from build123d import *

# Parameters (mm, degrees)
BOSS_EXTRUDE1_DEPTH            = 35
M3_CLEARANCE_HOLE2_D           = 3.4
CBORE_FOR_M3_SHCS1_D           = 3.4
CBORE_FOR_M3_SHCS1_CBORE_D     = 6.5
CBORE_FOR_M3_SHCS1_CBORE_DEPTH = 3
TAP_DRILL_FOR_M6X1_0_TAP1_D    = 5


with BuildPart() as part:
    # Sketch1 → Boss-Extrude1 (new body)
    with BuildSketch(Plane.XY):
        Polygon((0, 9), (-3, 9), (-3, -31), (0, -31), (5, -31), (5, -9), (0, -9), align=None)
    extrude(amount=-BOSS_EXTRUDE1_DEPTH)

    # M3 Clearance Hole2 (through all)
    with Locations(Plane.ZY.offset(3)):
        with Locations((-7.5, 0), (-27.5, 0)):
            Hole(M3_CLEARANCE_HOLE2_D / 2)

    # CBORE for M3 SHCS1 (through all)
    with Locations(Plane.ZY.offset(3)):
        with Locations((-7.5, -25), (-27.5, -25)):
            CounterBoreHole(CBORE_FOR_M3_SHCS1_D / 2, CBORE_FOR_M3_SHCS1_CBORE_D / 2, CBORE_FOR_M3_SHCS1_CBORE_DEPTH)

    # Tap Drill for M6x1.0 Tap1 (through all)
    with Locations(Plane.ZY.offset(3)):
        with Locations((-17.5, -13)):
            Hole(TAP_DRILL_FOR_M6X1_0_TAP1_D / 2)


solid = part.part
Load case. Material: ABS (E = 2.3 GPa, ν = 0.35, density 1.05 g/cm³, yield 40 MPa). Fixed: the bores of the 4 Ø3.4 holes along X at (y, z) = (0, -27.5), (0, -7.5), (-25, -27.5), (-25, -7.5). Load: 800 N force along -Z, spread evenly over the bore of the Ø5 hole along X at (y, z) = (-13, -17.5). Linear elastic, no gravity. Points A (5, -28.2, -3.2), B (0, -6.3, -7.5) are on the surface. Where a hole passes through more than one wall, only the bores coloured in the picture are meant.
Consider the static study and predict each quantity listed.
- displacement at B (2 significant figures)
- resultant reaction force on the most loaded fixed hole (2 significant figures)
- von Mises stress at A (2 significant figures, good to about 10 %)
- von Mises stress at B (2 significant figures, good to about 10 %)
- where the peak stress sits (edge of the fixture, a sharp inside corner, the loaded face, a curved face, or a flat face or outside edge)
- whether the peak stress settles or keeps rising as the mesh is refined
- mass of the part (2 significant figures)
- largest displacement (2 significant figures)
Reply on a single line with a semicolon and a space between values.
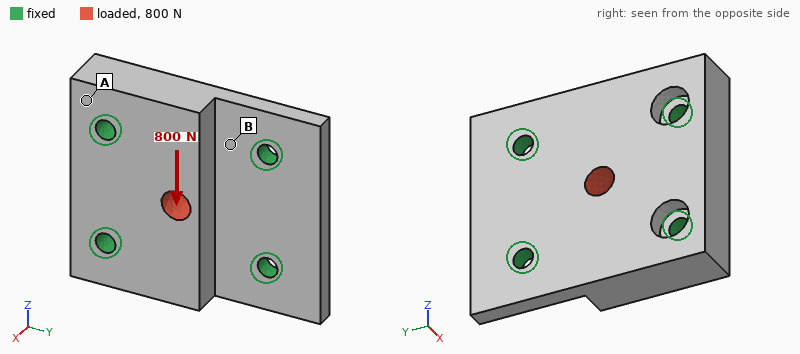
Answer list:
23 µm; 290 N; 1.4 MPa; 5.2 MPa; edge of the fixture; keeps rising; 7.9 g; 60 µm
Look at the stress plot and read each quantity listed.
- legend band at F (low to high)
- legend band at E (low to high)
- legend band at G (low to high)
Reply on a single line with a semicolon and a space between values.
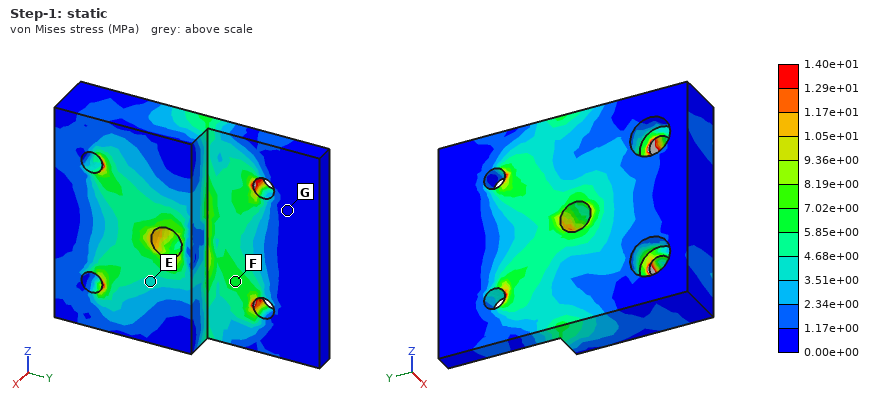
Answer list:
5.85e+00 to 7.02e+00 MPa; 3.51e+00 to 4.68e+00 MPa; 0.00e+00 to 1.17e+00 MPa
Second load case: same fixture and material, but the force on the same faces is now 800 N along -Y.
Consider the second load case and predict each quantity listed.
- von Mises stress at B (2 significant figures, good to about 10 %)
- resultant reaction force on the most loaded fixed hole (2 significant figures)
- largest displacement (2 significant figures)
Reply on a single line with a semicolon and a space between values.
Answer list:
3.8 MPa; 290 N; 78 µm
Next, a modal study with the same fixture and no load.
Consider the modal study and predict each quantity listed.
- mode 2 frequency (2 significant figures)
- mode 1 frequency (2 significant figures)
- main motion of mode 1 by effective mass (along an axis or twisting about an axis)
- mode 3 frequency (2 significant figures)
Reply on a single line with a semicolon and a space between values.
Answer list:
7700 Hz; 6600 Hz; along X; 7900 Hz
